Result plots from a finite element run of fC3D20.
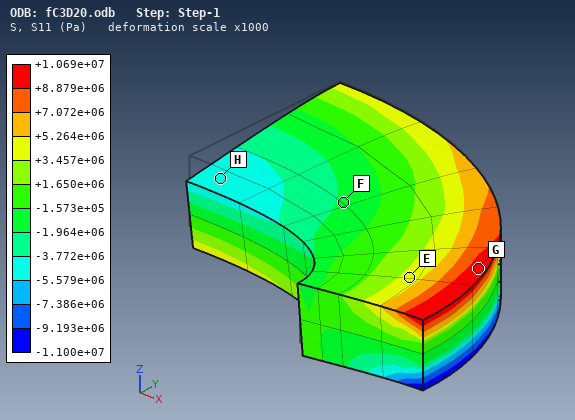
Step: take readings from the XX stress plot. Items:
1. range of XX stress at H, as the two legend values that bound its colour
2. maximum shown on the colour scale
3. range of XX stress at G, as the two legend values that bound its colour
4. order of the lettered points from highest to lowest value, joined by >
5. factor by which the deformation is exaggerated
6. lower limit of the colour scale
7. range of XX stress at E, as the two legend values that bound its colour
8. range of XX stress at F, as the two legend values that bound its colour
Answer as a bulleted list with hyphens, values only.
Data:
- -5.579e+06 to -3.772e+06 Pa
- +1.069e+07 Pa
- +8.879e+06 to +1.069e+07 Pa
- G > E > F > H
- 1000
- -1.100e+07 Pa
- +3.457e+06 to +5.264e+06 Pa
- -1.964e+06 to -1.573e+05 Pa
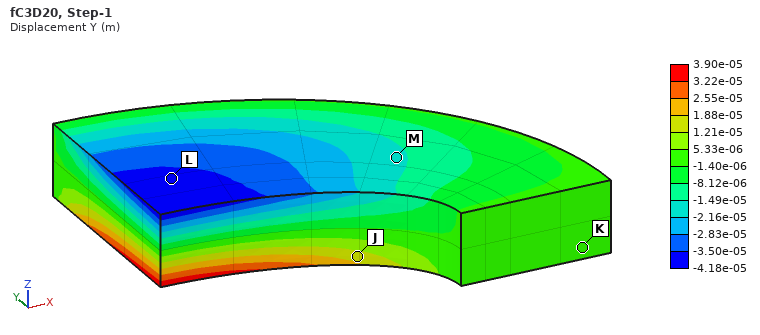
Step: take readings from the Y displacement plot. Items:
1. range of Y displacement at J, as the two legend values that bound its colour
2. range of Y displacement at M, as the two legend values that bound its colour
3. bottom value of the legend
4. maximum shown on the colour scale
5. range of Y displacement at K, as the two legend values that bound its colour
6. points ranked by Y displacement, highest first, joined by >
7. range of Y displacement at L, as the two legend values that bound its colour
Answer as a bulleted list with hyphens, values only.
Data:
- 1.21e-05 to 1.88e-05 m
- -2.16e-05 to -1.49e-05 m
- -4.18e-05 m
- 3.90e-05 m
- -1.40e-06 to 5.33e-06 m
- J > K > M > L
- -4.18e-05 to -3.50e-05 m
